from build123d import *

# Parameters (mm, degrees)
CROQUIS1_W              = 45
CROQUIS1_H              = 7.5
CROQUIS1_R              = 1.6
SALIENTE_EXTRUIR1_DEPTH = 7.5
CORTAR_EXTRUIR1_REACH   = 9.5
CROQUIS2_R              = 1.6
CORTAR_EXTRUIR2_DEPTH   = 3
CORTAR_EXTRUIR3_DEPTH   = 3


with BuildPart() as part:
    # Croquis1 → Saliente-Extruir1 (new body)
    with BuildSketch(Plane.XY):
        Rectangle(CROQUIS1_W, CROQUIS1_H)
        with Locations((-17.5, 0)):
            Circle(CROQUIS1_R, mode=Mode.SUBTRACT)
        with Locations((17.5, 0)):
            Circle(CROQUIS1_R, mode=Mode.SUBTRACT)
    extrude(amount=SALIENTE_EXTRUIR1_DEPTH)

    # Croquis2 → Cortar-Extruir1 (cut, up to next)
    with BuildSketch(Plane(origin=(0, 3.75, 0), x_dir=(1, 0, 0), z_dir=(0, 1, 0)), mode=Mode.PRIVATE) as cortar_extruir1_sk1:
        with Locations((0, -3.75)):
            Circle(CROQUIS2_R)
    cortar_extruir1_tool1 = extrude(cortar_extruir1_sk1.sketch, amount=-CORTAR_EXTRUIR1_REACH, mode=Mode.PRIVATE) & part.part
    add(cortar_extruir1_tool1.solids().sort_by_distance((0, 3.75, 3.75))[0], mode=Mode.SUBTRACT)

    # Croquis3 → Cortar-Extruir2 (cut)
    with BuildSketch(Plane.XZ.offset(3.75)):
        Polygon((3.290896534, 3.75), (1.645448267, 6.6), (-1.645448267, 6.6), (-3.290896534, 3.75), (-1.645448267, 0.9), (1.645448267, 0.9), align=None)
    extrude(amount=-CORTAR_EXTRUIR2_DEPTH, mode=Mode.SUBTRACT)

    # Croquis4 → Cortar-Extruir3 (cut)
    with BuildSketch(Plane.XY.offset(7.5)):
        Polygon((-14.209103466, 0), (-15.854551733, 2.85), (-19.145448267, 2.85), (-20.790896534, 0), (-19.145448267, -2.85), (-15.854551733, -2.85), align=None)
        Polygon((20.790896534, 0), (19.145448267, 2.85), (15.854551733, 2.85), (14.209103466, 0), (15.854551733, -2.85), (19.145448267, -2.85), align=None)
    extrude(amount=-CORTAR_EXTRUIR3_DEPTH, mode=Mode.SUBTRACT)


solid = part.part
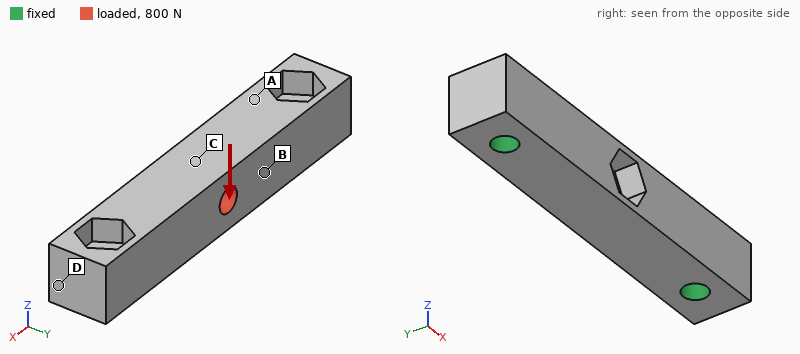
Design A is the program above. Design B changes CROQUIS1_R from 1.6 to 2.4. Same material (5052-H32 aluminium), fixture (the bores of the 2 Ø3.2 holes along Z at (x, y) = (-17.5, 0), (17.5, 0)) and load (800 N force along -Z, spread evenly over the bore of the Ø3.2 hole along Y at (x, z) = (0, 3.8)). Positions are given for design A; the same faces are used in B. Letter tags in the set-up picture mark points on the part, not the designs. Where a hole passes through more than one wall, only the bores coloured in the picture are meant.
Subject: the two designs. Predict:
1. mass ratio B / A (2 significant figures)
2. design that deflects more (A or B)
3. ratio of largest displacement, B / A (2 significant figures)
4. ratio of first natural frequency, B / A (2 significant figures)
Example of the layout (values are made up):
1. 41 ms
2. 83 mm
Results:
1. 0.96
2. A
3. 0.85
4. 1.2
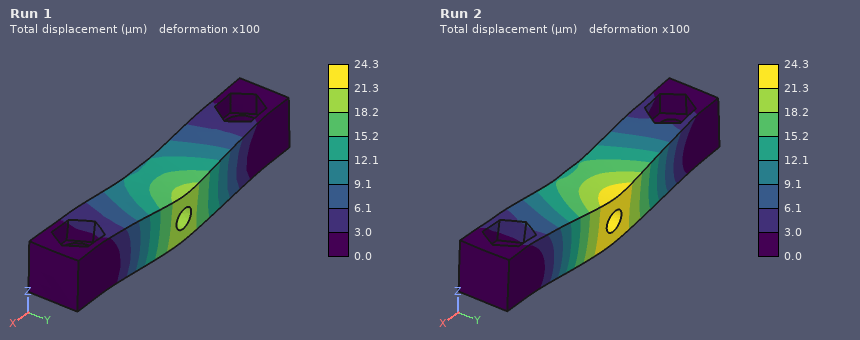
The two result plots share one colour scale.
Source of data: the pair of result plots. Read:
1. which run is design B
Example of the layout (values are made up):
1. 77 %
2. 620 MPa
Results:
1. Run 1
